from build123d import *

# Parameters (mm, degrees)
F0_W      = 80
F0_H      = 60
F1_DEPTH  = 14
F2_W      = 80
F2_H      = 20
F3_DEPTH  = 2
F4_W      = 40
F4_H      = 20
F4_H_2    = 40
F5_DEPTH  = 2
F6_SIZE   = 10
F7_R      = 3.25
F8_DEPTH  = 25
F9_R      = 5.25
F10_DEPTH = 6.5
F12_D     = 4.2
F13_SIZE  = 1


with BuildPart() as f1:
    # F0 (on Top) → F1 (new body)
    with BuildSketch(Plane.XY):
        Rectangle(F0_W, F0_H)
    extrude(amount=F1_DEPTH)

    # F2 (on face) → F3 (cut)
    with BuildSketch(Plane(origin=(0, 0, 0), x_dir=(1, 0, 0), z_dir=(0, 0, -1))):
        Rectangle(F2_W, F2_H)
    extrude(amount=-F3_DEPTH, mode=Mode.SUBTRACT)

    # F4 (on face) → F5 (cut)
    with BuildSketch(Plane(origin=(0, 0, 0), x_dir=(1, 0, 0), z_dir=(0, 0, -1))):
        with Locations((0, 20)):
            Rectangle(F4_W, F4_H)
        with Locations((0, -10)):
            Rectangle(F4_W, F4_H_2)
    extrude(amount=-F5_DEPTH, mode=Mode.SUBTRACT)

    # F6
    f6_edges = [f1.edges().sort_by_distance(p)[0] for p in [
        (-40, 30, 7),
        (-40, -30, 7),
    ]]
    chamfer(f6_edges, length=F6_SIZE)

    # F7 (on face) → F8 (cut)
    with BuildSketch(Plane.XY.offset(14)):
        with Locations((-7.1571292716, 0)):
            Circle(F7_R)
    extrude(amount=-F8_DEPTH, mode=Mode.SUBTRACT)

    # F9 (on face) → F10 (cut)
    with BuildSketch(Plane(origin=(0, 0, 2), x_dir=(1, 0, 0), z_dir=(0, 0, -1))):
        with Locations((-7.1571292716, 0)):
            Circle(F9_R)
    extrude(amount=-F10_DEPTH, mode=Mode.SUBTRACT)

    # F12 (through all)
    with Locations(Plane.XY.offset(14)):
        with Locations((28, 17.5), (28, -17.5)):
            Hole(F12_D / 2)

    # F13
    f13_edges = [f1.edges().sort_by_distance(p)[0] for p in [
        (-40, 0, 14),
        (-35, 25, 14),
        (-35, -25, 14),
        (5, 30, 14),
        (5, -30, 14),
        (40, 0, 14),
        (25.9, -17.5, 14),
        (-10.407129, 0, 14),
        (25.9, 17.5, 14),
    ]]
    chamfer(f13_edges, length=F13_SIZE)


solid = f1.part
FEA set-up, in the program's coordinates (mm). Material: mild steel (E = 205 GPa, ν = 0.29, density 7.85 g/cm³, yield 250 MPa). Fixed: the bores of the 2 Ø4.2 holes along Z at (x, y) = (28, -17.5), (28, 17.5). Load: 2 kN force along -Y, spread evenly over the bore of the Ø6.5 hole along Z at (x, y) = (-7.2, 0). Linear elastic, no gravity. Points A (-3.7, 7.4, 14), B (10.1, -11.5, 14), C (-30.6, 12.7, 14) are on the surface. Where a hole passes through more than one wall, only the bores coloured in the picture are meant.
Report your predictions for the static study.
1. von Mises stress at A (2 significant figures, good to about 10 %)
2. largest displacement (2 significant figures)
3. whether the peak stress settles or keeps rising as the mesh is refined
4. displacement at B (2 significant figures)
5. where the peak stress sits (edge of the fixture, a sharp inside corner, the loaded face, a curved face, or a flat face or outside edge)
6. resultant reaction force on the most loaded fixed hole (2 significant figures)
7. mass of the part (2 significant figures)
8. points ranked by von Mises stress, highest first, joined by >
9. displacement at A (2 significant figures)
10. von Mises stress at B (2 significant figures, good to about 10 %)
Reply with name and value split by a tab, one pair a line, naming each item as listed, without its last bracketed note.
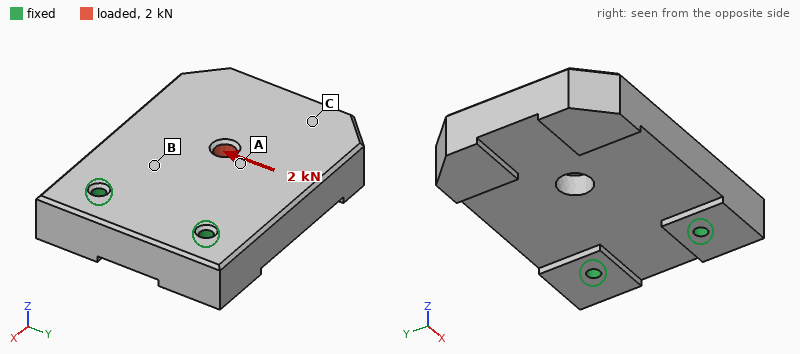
von Mises stress at A	12 MPa
largest displacement	4.5 µm
whether the peak stress settles or keeps rising as the mesh is refined	keeps rising
displacement at B	1.4 µm
where the peak stress sits	edge of the fixture
resultant reaction force on the most loaded fixed hole	2.1 kN
mass of the part	460 g
points ranked by von Mises stress, highest first, joined by >	A > B > C
displacement at A	2.7 µm
von Mises stress at B	8.7 MPa
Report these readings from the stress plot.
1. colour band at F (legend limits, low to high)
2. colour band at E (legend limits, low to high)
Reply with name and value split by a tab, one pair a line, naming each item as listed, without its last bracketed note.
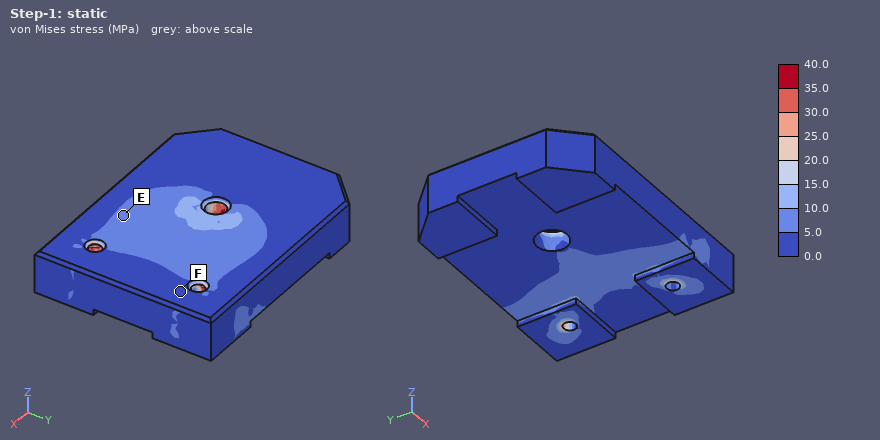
colour band at F	0.0 to 5.0 MPa
colour band at E	5.0 to 10.0 MPa
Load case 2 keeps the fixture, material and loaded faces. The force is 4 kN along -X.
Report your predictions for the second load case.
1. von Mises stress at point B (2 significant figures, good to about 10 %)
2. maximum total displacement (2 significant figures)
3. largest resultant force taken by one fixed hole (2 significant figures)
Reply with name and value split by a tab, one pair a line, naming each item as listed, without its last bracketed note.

von Mises stress at point B	14 MPa
maximum total displacement	13 µm
largest resultant force taken by one fixed hole	2.0 kN
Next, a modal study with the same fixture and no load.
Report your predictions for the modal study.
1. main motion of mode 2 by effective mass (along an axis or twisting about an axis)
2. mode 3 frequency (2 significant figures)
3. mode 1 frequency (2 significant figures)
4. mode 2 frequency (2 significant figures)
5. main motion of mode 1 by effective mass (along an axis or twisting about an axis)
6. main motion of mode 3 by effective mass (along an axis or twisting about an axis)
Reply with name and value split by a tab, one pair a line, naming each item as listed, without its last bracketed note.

main motion of mode 2 by effective mass	twisting about X
mode 3 frequency	6400 Hz
mode 1 frequency	2000 Hz
mode 2 frequency	5200 Hz
main motion of mode 1 by effective mass	along Z
main motion of mode 3 by effective mass	along Y
